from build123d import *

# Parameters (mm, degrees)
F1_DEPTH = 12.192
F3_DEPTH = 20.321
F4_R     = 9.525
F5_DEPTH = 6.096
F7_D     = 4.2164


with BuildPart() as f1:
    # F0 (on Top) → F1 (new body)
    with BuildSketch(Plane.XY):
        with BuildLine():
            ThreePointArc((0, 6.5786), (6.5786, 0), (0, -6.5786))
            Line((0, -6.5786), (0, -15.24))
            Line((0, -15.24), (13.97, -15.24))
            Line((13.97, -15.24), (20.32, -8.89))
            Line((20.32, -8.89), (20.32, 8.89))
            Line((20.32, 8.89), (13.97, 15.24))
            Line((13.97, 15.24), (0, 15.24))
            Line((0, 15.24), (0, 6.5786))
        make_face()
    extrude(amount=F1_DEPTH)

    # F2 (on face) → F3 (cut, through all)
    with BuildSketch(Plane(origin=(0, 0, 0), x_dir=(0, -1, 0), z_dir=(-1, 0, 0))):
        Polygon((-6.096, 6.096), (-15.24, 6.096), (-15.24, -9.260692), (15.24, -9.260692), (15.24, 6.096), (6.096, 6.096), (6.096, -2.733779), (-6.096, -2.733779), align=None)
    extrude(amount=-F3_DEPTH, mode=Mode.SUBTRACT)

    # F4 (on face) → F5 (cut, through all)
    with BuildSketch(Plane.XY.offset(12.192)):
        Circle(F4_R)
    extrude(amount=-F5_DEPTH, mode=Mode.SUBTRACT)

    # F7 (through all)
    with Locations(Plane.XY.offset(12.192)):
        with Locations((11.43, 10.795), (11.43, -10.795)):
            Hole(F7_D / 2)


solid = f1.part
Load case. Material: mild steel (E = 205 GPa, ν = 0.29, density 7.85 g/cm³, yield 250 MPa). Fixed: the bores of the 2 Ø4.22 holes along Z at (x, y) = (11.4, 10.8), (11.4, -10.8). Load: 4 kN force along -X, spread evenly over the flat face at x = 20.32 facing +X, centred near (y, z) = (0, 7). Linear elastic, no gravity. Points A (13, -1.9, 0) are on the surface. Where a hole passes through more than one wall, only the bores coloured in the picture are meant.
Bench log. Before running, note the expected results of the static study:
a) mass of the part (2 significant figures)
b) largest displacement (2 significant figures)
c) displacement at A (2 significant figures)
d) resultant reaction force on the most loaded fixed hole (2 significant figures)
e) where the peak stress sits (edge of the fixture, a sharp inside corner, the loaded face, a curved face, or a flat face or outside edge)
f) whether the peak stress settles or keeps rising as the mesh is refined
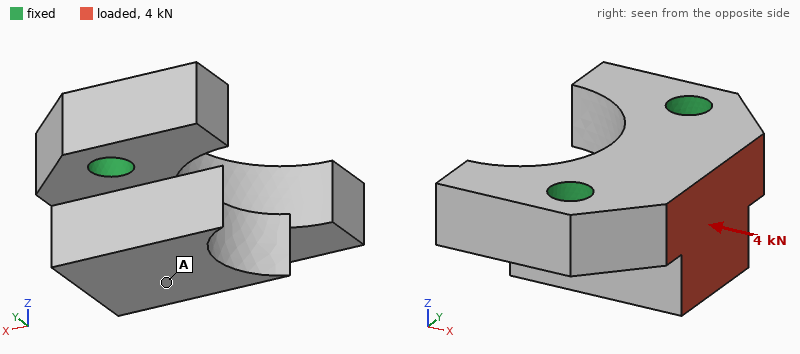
28 g
9.8 µm
7.9 µm
2.2 kN
edge of the fixture
keeps rising
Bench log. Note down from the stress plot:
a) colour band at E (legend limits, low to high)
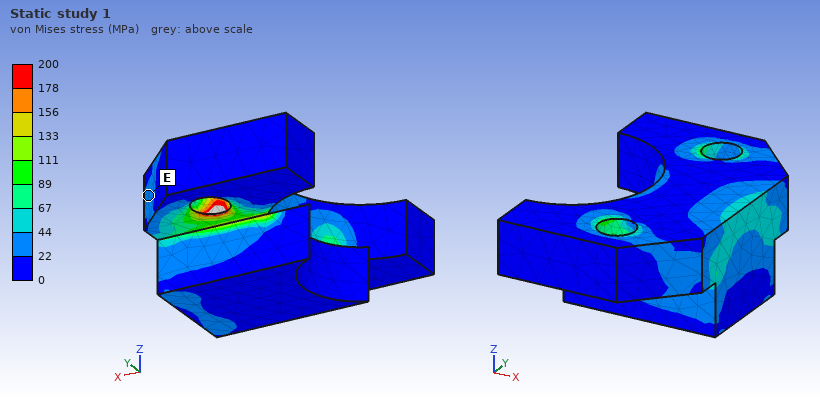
22 to 44 MPa
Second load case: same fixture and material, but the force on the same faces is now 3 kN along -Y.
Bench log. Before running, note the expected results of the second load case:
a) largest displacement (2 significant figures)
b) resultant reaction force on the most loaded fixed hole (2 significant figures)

4.7 µm
1.9 kN
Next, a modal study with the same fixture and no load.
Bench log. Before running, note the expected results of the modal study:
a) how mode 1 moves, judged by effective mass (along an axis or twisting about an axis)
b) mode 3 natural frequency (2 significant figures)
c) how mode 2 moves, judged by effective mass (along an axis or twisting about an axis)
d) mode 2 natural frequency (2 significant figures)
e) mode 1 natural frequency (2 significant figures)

along X
45 kHz
along Z
41 kHz
24 kHz
